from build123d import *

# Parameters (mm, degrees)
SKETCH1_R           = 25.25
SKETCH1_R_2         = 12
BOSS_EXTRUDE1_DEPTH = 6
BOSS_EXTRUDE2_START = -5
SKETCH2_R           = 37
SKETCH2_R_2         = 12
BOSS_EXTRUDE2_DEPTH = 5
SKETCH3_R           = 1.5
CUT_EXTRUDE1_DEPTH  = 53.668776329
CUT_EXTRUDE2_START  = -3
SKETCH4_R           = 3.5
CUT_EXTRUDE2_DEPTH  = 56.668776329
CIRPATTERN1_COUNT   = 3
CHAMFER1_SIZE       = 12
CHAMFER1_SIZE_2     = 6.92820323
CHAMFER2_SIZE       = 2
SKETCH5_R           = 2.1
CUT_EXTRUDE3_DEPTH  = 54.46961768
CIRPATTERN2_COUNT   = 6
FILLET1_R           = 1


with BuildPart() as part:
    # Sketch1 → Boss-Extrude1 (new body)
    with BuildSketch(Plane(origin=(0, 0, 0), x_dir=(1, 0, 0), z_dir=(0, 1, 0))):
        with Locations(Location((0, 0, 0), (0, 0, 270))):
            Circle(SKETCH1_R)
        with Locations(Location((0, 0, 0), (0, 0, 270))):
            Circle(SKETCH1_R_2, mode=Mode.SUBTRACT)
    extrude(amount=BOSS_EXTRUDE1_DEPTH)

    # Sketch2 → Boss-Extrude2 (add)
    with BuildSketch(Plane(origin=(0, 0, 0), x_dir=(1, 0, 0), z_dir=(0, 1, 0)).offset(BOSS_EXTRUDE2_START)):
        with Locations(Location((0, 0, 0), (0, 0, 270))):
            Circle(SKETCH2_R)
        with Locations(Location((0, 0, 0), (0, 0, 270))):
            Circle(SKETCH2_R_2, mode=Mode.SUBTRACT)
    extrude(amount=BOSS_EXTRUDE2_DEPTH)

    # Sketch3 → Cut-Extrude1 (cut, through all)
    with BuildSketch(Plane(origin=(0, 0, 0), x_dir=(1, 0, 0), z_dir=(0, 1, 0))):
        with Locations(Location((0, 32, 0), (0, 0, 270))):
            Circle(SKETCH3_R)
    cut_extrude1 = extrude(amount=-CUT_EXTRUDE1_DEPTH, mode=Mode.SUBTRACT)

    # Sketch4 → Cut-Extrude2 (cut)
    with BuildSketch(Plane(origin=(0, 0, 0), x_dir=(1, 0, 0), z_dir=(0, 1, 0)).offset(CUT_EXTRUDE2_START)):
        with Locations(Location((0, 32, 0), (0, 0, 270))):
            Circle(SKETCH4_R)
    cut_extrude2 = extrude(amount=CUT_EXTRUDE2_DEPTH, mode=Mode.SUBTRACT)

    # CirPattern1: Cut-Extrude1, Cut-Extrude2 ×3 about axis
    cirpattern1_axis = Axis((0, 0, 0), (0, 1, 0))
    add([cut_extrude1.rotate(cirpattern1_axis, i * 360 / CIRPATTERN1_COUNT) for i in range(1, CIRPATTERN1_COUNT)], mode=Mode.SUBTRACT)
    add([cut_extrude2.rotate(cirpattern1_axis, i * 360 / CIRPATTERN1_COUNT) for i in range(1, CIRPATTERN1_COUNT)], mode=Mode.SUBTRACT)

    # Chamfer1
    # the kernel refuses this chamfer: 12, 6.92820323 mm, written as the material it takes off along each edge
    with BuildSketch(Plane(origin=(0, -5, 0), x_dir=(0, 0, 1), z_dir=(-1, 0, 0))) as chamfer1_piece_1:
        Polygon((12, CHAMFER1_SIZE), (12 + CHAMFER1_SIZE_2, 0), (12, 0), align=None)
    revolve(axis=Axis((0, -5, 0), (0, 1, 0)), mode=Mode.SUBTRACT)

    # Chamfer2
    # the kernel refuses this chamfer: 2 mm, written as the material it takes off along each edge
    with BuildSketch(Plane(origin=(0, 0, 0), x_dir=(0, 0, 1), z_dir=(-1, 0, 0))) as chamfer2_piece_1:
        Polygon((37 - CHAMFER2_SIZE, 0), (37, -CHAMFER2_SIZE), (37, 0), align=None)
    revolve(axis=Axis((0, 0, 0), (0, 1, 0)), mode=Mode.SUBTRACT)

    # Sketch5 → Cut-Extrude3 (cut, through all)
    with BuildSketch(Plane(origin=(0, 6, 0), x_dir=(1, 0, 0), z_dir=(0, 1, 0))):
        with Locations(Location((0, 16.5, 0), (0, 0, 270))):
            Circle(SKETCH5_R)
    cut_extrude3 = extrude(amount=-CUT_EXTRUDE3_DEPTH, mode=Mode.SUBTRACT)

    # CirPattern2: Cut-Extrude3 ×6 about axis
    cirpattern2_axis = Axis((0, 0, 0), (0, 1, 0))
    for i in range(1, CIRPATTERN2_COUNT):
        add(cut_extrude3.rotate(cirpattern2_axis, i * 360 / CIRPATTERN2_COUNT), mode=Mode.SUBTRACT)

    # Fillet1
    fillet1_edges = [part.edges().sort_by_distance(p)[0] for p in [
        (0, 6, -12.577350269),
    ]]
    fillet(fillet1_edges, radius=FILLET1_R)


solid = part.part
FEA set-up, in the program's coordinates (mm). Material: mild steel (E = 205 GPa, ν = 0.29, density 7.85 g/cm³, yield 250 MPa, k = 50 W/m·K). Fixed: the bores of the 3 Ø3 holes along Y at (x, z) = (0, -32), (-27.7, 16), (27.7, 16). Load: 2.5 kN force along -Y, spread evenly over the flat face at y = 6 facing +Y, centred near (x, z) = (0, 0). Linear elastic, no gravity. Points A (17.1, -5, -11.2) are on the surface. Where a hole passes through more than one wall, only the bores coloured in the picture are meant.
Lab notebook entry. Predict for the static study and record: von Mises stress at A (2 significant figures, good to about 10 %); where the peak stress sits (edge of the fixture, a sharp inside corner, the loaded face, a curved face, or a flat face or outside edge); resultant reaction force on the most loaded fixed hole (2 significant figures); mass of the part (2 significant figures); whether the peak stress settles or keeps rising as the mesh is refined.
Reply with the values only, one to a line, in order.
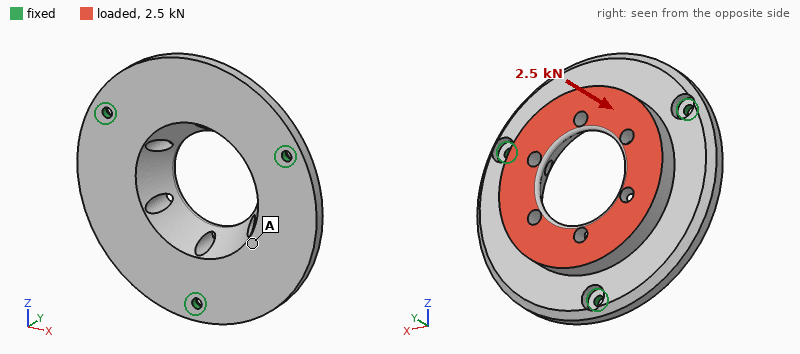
15 MPa
edge of the fixture
1.2 kN
180 g
keeps rising
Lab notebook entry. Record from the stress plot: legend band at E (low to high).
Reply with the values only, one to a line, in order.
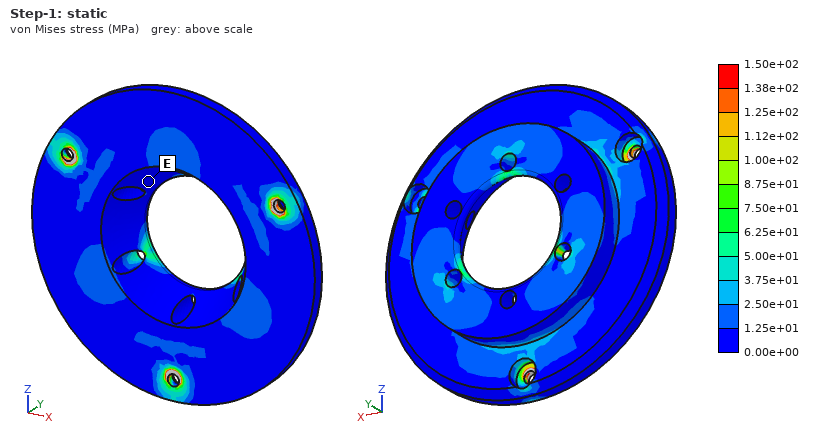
0.00e+00 to 1.25e+01 MPa
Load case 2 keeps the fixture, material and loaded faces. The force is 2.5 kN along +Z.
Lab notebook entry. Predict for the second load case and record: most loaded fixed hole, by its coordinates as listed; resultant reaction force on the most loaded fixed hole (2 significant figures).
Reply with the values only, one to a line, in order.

(0, -32)
1.1 kN
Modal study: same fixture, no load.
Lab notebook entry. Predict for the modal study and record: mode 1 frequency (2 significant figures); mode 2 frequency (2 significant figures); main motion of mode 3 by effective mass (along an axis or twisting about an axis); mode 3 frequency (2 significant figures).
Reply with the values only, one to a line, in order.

5600 Hz
5600 Hz
along Y
6800 Hz
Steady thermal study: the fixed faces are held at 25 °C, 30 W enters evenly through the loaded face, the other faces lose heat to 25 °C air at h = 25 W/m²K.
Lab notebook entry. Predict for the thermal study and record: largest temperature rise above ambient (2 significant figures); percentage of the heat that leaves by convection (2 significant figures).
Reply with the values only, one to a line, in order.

32 K
19 %
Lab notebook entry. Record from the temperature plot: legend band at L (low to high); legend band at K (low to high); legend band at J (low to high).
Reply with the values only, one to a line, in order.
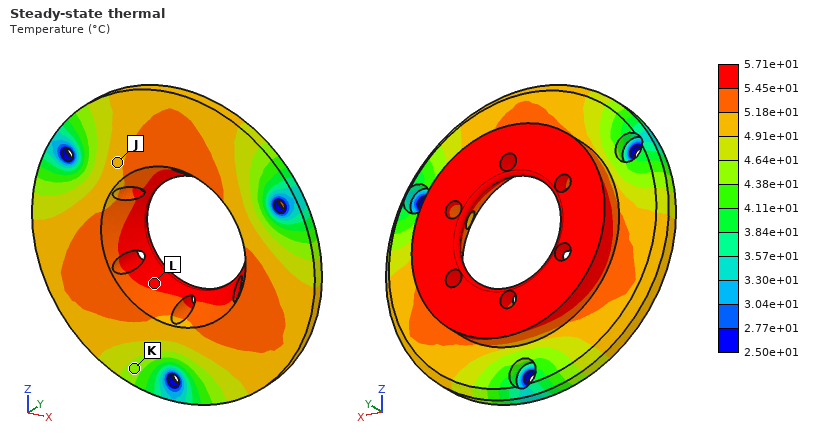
5.45e+01 to 5.71e+01 °C
4.38e+01 to 4.64e+01 °C
4.91e+01 to 5.18e+01 °C
